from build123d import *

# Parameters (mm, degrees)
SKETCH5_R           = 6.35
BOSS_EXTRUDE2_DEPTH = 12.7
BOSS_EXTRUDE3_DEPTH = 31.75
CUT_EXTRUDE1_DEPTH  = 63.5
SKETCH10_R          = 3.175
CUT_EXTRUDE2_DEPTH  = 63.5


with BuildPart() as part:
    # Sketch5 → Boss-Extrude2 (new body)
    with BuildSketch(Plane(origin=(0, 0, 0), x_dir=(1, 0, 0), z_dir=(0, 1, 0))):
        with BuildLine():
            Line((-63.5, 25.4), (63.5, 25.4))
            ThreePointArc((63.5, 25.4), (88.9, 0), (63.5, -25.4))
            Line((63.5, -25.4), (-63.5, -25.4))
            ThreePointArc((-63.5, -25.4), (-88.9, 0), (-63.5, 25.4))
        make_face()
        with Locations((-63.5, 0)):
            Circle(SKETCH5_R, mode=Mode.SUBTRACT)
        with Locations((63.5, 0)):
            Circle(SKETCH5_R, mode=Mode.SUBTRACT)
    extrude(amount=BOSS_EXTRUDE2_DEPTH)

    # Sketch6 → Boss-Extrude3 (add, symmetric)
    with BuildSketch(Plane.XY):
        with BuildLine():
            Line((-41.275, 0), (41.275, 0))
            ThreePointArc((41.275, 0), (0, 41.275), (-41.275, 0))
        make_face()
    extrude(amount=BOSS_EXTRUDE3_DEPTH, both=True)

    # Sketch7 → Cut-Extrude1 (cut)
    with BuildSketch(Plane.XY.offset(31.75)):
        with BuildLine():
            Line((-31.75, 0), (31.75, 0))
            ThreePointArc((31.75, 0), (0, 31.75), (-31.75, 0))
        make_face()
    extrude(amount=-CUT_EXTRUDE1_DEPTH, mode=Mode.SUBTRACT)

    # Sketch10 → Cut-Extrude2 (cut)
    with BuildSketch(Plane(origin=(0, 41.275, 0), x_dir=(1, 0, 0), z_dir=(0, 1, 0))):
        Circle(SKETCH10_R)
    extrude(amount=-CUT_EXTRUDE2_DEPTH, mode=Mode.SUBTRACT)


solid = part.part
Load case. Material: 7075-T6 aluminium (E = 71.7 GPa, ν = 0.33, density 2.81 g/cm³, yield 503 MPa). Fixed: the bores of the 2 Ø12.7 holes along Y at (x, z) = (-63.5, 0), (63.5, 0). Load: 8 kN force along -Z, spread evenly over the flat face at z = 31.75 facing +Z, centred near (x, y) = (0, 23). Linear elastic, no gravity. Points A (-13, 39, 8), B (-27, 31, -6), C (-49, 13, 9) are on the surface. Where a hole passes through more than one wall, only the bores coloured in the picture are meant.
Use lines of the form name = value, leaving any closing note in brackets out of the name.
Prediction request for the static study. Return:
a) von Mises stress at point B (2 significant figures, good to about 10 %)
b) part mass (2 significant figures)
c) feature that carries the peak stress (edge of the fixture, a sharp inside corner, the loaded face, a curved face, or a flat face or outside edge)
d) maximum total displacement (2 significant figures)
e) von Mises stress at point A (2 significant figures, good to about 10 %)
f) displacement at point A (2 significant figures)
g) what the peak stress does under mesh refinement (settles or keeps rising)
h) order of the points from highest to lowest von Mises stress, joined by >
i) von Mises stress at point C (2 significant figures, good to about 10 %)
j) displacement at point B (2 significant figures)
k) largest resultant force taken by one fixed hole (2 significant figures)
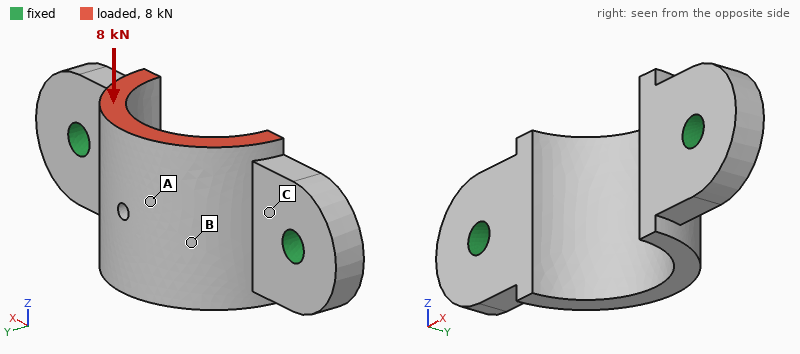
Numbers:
von Mises stress at point B = 19 MPa
part mass = 340 g
feature that carries the peak stress = edge of the fixture
maximum total displacement = 0.14 mm
von Mises stress at point A = 11 MPa
displacement at point A = 0.11 mm
what the peak stress does under mesh refinement = keeps rising
order of the points from highest to lowest von Mises stress, joined by > = C > B > A
von Mises stress at point C = 49 MPa
displacement at point B = 0.083 mm
largest resultant force taken by one fixed hole = 4.0 kN
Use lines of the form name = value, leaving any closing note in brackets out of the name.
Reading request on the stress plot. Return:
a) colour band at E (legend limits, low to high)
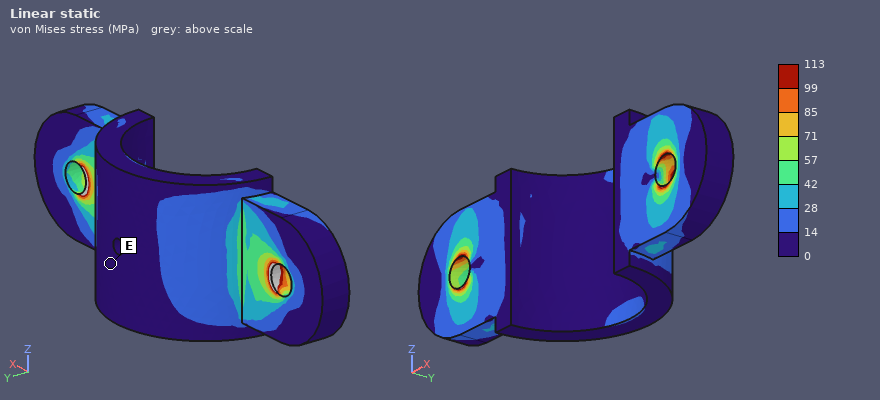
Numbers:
colour band at E = 0 to 14 MPa
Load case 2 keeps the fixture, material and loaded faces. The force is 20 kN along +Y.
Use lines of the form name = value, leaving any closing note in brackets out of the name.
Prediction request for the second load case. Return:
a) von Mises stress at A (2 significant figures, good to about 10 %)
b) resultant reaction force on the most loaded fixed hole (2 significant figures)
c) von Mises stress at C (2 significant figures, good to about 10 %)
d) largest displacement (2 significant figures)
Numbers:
von Mises stress at A = 44 MPa
resultant reaction force on the most loaded fixed hole = 13 kN
von Mises stress at C = 160 MPa
largest displacement = 0.54 mm
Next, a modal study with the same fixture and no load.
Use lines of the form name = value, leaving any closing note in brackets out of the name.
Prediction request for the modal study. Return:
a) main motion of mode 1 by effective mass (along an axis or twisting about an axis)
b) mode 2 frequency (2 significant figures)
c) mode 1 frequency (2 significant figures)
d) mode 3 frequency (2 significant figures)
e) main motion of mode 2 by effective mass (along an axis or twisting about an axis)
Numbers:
main motion of mode 1 by effective mass = along Z
mode 2 frequency = 5700 Hz
mode 1 frequency = 3000 Hz
mode 3 frequency = 6300 Hz
main motion of mode 2 by effective mass = along Y
